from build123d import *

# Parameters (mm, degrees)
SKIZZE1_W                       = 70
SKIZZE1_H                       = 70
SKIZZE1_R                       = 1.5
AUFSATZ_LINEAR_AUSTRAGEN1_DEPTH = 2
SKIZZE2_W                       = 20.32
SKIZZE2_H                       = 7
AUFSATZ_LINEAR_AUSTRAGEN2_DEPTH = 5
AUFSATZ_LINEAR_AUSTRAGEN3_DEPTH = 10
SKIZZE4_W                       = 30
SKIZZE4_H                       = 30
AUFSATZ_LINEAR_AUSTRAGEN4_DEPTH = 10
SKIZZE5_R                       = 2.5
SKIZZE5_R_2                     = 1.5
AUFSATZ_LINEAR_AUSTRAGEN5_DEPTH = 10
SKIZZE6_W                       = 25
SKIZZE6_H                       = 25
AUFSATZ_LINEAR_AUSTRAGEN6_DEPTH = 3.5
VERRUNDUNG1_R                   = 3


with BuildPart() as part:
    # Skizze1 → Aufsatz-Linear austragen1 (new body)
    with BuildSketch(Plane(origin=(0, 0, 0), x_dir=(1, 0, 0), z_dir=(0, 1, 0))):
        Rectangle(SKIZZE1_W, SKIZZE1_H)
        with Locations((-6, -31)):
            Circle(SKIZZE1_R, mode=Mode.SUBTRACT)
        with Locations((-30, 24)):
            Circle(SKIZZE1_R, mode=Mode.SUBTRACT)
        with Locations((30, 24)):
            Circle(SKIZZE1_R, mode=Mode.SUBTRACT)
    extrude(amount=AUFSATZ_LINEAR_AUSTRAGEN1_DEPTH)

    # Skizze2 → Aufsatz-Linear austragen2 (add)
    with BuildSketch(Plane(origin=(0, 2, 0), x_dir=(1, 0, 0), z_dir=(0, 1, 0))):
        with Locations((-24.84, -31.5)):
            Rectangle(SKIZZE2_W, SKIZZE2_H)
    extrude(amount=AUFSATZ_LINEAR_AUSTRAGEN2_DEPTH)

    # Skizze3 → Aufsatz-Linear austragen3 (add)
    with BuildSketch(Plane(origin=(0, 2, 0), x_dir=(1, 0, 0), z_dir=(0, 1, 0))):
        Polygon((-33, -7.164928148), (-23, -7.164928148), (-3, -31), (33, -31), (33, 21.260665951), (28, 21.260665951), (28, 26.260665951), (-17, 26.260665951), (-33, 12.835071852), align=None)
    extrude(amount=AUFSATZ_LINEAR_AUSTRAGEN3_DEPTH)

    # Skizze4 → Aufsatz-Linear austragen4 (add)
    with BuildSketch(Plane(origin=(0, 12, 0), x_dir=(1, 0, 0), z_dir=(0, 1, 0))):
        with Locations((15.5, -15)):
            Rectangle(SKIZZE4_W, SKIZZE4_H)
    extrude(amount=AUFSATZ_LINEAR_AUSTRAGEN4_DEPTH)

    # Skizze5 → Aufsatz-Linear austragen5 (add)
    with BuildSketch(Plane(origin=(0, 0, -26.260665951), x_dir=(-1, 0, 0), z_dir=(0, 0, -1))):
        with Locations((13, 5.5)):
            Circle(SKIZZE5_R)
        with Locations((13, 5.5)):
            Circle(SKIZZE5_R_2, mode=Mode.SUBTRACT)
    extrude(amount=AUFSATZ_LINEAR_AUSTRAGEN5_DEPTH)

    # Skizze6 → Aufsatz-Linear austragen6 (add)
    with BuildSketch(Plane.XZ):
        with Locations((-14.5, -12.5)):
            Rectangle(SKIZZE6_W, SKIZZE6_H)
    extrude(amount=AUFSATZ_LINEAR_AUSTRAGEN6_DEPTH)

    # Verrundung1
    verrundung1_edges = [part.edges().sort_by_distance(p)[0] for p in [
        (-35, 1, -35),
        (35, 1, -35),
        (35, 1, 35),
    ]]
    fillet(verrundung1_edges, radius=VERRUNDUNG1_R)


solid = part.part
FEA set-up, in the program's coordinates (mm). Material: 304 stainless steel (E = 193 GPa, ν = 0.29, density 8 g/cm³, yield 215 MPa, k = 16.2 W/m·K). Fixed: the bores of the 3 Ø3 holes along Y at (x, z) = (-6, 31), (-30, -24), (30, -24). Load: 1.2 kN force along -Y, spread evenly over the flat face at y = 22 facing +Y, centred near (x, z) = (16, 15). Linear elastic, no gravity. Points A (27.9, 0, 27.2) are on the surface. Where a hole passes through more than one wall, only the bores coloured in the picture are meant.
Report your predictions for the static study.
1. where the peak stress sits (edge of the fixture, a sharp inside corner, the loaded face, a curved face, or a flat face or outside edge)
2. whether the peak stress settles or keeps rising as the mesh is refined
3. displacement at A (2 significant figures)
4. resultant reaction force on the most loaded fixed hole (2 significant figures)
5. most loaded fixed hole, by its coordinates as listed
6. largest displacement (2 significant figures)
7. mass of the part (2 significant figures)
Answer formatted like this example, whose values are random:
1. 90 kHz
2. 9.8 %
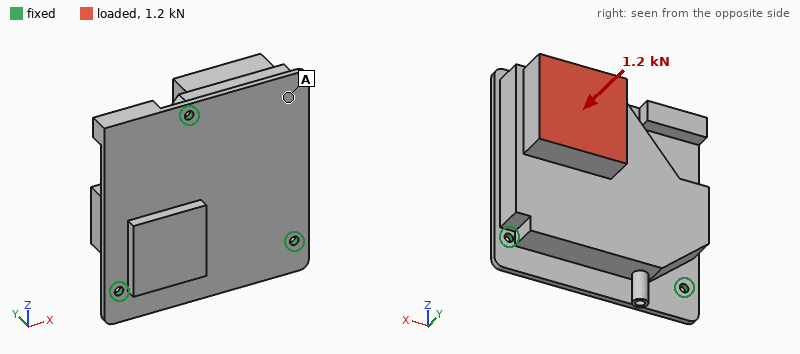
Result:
1. edge of the fixture
2. keeps rising
3. 13 µm
4. 1.1 kN
5. (-6, 31)
6. 15 µm
7. 430 g
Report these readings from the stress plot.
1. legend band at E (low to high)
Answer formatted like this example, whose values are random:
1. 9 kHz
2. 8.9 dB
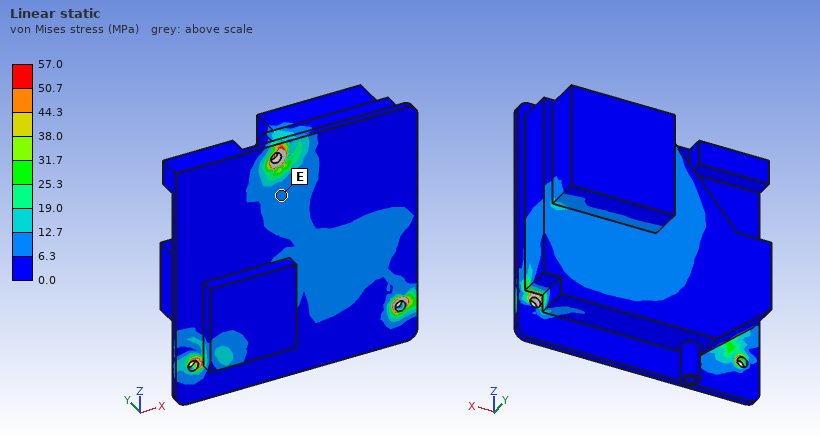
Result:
1. 6.3 to 12.7 MPa
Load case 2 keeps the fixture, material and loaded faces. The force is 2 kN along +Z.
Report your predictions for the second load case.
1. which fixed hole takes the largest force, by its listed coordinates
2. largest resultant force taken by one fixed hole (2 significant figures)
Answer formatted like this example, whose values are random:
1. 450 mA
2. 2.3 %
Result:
1. (-6, 31)
2. 1.2 kN
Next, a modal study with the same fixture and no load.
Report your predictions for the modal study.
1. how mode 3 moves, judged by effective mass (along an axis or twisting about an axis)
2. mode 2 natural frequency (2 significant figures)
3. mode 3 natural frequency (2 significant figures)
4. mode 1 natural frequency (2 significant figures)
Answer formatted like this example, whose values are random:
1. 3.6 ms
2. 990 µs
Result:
1. along Y
2. 3700 Hz
3. 5000 Hz
4. 2800 Hz
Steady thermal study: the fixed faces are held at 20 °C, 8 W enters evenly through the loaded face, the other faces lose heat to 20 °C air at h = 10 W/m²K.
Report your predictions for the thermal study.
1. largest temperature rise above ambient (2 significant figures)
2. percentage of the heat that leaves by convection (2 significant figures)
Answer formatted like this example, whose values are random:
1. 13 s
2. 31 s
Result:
1. 38 K
2. 35 %
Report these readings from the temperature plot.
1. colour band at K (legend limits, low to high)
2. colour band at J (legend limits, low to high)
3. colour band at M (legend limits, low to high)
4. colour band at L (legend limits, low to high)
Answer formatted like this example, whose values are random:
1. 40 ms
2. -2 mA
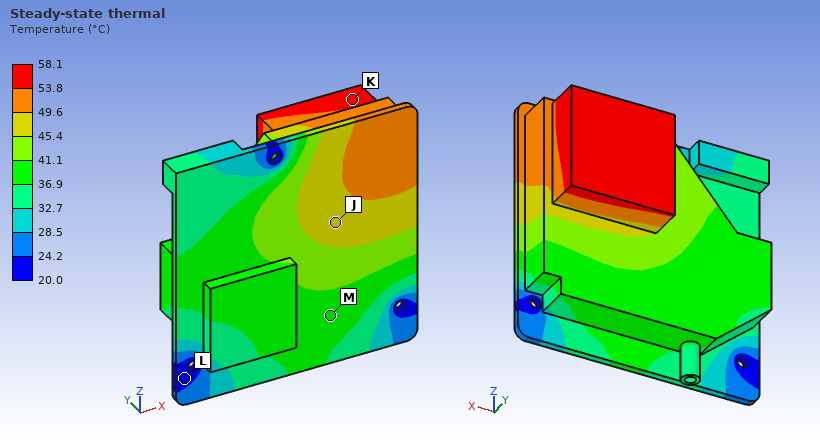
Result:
1. 53.8 to 58.1 °C
2. 45.4 to 49.6 °C
3. 36.9 to 41.1 °C
4. 20.0 to 24.2 °C
